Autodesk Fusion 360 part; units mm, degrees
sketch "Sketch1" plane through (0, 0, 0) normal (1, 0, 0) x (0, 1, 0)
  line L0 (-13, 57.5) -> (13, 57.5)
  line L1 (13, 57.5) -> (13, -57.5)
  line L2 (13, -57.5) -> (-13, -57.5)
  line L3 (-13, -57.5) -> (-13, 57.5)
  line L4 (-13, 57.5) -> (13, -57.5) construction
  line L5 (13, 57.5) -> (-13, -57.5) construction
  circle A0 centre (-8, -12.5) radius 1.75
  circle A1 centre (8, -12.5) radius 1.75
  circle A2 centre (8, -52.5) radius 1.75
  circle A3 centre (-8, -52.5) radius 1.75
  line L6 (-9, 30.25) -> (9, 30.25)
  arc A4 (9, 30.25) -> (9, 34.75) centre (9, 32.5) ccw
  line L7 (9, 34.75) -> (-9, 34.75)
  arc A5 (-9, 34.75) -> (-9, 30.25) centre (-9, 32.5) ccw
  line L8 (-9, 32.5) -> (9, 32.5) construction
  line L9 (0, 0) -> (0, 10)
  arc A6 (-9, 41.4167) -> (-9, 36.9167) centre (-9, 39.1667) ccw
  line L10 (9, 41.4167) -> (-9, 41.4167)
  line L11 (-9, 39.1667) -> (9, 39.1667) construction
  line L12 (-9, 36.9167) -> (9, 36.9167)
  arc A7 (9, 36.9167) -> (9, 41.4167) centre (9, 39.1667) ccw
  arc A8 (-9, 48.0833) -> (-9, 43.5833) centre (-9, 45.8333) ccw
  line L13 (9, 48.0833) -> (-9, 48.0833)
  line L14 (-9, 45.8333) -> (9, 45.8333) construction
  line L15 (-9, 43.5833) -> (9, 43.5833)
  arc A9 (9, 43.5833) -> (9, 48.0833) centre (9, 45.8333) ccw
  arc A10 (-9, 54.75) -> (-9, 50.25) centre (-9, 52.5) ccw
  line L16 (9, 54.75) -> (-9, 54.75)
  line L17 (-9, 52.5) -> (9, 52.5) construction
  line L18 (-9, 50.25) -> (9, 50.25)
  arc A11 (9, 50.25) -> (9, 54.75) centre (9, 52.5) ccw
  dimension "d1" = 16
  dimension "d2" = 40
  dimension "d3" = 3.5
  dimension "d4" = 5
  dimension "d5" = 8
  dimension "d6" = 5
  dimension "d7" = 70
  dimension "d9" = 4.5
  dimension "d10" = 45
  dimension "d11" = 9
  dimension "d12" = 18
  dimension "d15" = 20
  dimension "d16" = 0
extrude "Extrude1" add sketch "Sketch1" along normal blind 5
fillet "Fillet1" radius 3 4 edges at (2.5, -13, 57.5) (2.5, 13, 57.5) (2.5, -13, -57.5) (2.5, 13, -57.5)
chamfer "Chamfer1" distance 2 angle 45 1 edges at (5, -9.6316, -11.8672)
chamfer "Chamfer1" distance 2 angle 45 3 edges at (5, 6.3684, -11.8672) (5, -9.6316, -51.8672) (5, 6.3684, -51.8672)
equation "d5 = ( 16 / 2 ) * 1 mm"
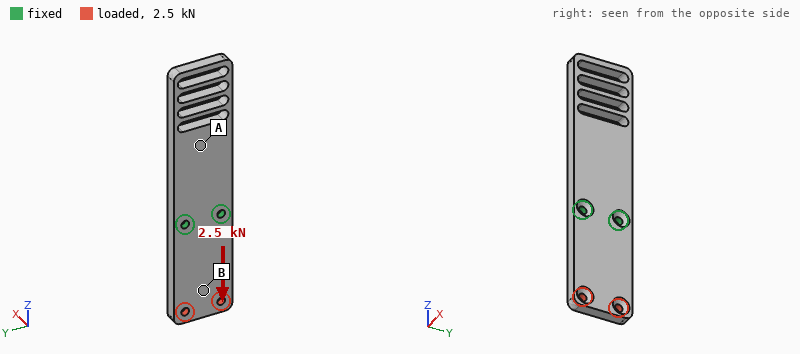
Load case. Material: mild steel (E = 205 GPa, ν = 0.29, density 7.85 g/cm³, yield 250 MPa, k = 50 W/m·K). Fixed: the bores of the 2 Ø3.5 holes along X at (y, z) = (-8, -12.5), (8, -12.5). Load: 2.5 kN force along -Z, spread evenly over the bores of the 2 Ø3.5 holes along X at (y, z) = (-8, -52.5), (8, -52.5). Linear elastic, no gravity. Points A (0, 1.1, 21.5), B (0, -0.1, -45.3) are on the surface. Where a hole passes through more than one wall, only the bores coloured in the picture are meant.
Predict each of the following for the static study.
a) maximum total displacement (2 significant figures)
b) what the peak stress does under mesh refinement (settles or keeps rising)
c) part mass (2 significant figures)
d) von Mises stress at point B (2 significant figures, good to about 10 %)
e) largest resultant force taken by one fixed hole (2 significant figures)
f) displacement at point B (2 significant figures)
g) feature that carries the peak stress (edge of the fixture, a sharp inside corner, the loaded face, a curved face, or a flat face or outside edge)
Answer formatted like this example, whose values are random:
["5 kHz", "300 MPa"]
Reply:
["43 µm", "keeps rising", "99 g", "36 MPa", "1.3 kN", "23 µm", "edge of the fixture"]
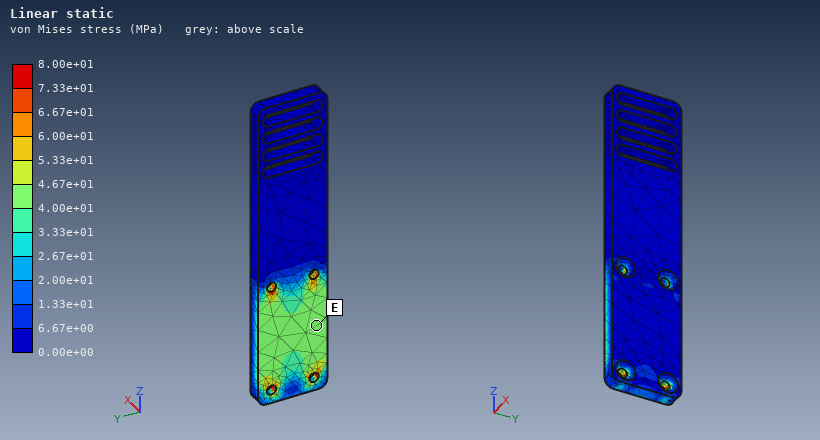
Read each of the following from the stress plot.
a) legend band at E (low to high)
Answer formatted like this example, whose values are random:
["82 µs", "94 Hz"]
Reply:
["4.00e+01 to 4.67e+01 MPa"]
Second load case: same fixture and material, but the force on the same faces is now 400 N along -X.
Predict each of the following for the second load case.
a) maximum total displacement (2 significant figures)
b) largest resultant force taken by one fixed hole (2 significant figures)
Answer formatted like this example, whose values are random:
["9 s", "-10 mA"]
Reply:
["0.22 mm", "250 N"]
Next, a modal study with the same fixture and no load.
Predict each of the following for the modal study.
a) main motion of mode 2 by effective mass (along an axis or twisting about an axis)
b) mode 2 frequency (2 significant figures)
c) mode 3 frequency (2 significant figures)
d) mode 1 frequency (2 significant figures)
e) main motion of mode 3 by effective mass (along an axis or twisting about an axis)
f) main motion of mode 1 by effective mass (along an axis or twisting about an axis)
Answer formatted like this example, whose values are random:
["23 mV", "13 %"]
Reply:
["along X", "1900 Hz", "3400 Hz", "990 Hz", "along Y", "along X"]
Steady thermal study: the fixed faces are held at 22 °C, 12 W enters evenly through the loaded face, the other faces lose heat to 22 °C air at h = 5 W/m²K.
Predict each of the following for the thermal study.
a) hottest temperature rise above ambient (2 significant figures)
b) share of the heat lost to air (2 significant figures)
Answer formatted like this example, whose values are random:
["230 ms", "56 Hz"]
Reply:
["81 K", "5.6 %"]
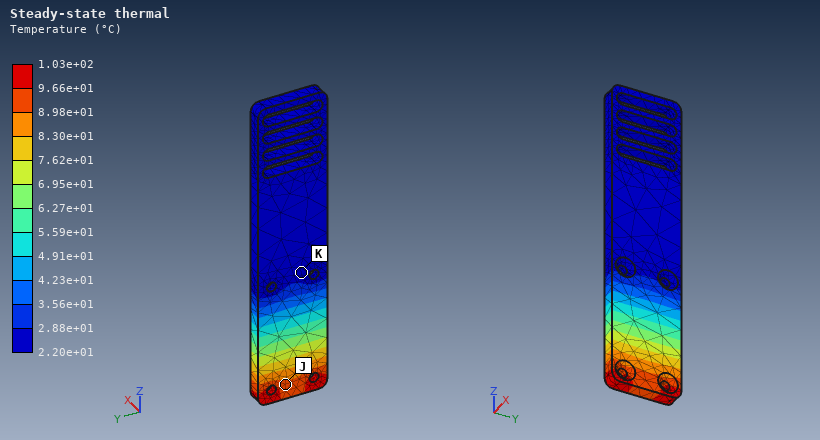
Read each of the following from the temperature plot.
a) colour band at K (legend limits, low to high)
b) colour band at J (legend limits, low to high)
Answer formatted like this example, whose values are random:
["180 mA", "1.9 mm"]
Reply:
["2.20e+01 to 2.88e+01 °C", "8.98e+01 to 9.66e+01 °C"]
